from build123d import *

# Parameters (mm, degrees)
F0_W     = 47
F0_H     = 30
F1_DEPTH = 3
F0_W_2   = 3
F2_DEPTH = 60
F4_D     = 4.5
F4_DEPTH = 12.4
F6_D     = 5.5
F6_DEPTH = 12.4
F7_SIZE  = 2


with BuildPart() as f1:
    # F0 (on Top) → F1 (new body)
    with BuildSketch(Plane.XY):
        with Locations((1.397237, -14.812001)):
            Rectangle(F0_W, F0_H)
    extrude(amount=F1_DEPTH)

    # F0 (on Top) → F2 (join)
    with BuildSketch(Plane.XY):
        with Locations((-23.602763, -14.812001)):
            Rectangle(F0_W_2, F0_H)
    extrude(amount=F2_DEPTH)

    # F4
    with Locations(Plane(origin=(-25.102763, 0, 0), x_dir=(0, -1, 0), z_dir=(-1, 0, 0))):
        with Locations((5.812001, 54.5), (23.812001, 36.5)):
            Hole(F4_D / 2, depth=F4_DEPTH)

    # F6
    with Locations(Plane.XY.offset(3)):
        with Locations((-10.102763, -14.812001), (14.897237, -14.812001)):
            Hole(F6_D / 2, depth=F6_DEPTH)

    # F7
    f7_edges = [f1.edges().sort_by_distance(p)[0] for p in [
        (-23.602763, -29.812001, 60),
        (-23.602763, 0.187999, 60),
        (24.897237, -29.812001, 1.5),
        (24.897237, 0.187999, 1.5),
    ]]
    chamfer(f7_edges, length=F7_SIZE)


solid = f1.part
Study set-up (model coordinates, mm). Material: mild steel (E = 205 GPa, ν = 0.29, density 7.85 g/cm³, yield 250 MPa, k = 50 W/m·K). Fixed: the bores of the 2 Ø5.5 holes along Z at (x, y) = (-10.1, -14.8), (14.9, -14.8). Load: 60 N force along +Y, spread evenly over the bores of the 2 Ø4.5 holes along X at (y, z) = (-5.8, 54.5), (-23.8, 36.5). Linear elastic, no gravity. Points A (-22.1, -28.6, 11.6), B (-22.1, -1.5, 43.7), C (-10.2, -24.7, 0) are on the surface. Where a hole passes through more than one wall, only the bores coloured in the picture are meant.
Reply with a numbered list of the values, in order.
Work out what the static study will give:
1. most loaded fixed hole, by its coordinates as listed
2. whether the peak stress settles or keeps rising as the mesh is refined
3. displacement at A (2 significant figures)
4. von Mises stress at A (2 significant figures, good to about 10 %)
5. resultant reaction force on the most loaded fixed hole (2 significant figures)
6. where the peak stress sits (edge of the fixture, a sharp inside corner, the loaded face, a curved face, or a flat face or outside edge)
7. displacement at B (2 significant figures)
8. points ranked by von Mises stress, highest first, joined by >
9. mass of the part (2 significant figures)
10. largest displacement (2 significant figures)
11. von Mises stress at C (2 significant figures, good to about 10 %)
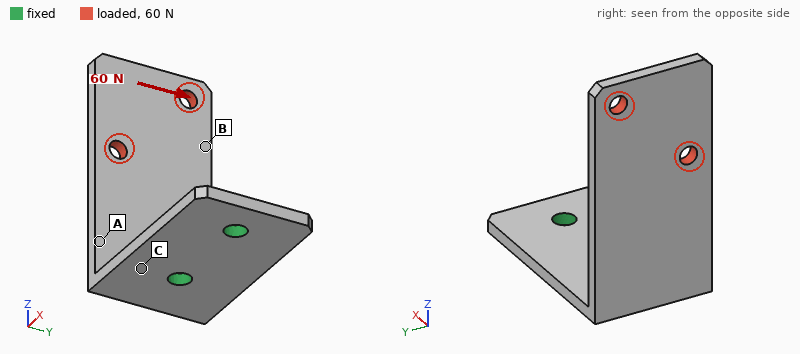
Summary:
1. (-10.1, -14.8)
2. keeps rising
3. 22 µm
4. 13 MPa
5. 82 N
6. edge of the fixture
7. 57 µm
8. C > A > B
9. 74 g
10. 77 µm
11. 27 MPa
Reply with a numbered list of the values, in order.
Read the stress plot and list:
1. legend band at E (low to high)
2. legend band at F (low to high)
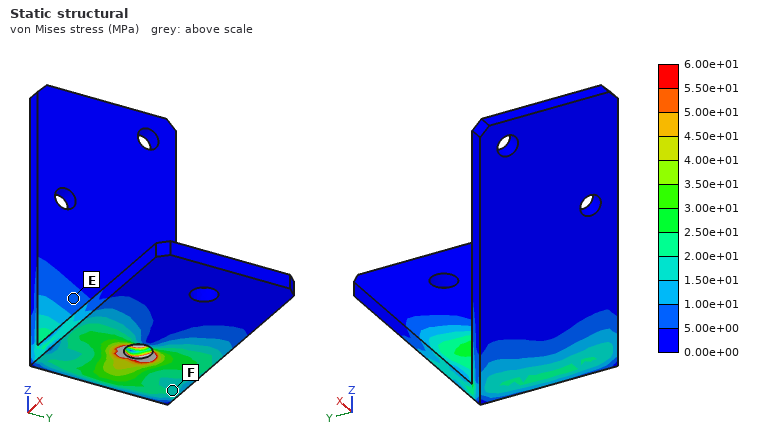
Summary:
1. 5.00e+00 to 1.00e+01 MPa
2. 1.50e+01 to 2.00e+01 MPa
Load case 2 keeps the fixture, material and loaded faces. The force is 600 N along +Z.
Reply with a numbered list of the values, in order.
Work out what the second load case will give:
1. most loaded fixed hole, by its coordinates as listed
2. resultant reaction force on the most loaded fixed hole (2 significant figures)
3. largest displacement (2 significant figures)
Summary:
1. (-10.1, -14.8)
2. 660 N
3. 0.22 mm
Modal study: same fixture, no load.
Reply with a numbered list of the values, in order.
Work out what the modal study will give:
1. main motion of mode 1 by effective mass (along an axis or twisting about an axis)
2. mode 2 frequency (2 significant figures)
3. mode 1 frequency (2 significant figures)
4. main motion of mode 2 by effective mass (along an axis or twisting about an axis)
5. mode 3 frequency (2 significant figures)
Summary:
1. along X
2. 1000 Hz
3. 550 Hz
4. along Y
5. 2900 Hz
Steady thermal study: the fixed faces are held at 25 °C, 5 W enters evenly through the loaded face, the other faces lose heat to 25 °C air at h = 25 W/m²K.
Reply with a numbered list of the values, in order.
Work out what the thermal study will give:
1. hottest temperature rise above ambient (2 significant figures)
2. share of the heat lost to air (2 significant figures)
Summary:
1. 44 K
2. 52 %
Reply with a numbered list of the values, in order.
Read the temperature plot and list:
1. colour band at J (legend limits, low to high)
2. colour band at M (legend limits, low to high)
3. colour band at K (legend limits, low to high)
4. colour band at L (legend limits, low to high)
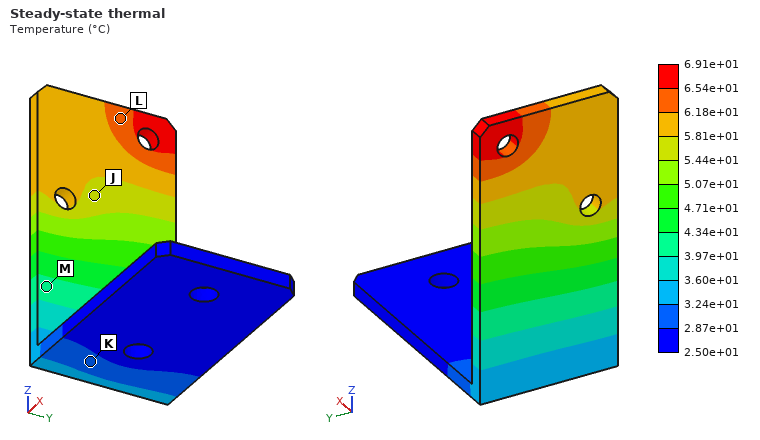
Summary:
1. 5.44e+01 to 5.81e+01 °C
2. 3.97e+01 to 4.34e+01 °C
3. 2.87e+01 to 3.24e+01 °C
4. 6.18e+01 to 6.54e+01 °C
